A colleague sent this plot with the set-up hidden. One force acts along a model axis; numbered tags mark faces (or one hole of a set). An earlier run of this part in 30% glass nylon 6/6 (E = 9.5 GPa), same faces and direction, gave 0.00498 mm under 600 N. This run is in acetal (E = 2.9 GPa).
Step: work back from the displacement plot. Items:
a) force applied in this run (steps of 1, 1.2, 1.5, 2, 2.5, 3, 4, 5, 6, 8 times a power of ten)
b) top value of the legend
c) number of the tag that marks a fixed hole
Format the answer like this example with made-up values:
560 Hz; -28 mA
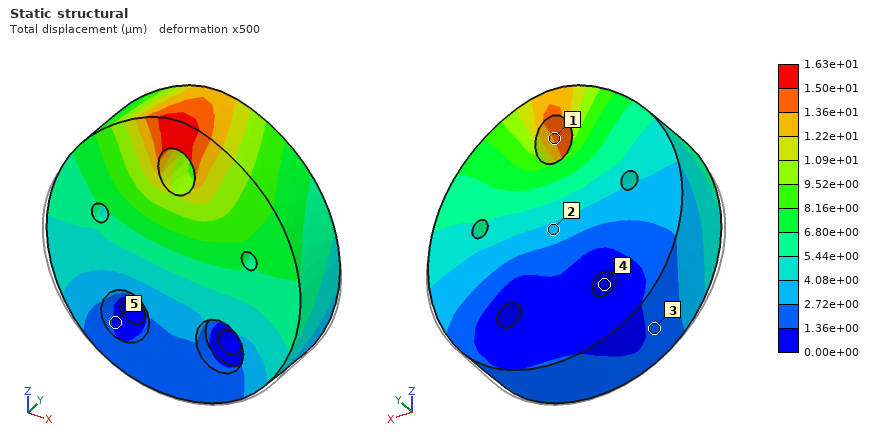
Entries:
600 N; 1.63e+01 µm; 4
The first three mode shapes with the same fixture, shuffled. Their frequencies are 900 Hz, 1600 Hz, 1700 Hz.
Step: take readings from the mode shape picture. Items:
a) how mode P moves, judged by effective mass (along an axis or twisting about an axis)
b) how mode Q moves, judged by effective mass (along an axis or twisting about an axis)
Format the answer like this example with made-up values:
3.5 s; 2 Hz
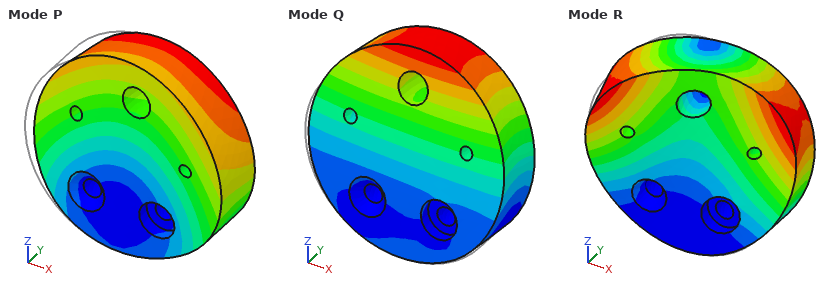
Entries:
along X; along Y
